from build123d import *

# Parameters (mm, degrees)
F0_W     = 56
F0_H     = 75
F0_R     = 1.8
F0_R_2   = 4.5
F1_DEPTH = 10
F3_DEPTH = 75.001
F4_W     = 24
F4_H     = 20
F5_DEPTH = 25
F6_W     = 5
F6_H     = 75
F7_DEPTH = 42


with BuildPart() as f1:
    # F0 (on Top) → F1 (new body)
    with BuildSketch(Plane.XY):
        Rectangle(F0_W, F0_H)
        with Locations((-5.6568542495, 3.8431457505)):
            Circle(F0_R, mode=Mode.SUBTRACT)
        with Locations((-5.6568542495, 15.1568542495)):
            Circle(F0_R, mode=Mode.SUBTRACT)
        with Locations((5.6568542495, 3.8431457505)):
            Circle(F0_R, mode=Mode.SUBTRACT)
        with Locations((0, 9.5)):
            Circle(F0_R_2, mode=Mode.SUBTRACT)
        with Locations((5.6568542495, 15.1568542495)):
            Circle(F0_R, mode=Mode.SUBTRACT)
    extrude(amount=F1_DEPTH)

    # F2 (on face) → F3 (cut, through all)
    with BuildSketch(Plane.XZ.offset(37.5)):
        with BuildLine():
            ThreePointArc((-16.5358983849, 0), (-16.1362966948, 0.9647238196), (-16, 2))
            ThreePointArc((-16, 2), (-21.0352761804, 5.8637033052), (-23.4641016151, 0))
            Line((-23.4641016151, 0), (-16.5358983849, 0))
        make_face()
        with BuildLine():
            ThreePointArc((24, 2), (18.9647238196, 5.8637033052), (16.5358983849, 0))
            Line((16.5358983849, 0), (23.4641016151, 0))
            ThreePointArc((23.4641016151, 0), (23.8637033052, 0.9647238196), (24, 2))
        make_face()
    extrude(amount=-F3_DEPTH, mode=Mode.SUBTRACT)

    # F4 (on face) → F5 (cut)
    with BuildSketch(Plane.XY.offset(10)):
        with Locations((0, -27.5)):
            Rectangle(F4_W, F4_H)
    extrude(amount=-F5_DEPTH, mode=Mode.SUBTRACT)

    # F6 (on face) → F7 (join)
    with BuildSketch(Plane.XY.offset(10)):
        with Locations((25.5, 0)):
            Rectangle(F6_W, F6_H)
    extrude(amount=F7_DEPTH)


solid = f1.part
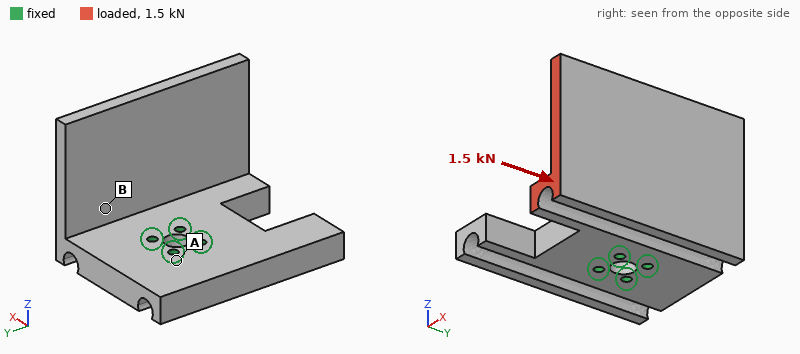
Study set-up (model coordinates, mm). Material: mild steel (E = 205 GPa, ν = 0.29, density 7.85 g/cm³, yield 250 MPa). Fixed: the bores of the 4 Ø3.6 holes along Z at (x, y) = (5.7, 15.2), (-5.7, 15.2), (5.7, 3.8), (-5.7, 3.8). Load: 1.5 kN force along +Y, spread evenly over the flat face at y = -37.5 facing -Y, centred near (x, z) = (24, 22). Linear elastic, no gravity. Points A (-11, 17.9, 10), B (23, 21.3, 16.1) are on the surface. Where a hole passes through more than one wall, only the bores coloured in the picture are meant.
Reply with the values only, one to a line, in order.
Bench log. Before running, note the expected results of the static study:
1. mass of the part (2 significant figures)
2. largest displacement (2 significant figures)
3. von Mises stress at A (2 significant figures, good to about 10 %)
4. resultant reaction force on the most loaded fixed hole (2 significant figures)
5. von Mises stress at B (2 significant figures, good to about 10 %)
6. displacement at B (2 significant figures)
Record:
360 g
35 µm
4.8 MPa
1.6 kN
16 MPa
8.1 µm
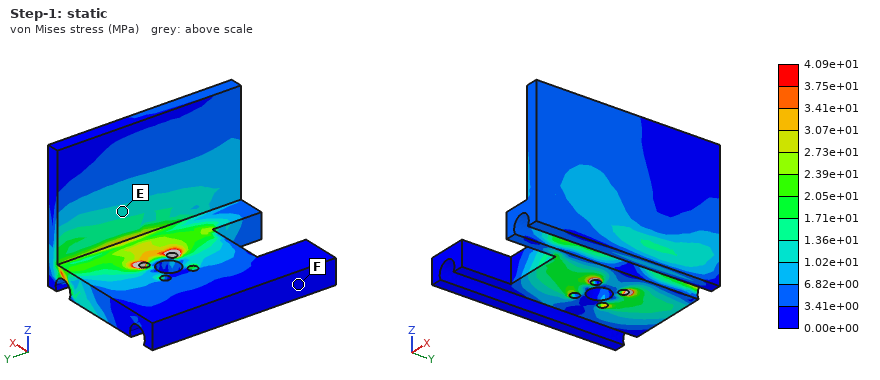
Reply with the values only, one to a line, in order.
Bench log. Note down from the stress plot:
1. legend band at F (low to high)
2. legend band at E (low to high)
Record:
0.00e+00 to 3.41e+00 MPa
1.02e+01 to 1.36e+01 MPa
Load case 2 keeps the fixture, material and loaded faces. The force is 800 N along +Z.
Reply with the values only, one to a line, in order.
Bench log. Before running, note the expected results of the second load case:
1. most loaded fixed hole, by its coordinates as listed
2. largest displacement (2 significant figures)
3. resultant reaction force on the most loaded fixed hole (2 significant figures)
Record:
(5.7, 3.8)
71 µm
1.8 kN
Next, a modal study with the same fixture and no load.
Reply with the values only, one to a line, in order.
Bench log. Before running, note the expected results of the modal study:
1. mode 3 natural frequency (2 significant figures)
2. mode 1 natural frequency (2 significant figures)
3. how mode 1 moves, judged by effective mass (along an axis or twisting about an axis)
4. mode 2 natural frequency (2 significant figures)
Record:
3200 Hz
1300 Hz
along X
2400 Hz
